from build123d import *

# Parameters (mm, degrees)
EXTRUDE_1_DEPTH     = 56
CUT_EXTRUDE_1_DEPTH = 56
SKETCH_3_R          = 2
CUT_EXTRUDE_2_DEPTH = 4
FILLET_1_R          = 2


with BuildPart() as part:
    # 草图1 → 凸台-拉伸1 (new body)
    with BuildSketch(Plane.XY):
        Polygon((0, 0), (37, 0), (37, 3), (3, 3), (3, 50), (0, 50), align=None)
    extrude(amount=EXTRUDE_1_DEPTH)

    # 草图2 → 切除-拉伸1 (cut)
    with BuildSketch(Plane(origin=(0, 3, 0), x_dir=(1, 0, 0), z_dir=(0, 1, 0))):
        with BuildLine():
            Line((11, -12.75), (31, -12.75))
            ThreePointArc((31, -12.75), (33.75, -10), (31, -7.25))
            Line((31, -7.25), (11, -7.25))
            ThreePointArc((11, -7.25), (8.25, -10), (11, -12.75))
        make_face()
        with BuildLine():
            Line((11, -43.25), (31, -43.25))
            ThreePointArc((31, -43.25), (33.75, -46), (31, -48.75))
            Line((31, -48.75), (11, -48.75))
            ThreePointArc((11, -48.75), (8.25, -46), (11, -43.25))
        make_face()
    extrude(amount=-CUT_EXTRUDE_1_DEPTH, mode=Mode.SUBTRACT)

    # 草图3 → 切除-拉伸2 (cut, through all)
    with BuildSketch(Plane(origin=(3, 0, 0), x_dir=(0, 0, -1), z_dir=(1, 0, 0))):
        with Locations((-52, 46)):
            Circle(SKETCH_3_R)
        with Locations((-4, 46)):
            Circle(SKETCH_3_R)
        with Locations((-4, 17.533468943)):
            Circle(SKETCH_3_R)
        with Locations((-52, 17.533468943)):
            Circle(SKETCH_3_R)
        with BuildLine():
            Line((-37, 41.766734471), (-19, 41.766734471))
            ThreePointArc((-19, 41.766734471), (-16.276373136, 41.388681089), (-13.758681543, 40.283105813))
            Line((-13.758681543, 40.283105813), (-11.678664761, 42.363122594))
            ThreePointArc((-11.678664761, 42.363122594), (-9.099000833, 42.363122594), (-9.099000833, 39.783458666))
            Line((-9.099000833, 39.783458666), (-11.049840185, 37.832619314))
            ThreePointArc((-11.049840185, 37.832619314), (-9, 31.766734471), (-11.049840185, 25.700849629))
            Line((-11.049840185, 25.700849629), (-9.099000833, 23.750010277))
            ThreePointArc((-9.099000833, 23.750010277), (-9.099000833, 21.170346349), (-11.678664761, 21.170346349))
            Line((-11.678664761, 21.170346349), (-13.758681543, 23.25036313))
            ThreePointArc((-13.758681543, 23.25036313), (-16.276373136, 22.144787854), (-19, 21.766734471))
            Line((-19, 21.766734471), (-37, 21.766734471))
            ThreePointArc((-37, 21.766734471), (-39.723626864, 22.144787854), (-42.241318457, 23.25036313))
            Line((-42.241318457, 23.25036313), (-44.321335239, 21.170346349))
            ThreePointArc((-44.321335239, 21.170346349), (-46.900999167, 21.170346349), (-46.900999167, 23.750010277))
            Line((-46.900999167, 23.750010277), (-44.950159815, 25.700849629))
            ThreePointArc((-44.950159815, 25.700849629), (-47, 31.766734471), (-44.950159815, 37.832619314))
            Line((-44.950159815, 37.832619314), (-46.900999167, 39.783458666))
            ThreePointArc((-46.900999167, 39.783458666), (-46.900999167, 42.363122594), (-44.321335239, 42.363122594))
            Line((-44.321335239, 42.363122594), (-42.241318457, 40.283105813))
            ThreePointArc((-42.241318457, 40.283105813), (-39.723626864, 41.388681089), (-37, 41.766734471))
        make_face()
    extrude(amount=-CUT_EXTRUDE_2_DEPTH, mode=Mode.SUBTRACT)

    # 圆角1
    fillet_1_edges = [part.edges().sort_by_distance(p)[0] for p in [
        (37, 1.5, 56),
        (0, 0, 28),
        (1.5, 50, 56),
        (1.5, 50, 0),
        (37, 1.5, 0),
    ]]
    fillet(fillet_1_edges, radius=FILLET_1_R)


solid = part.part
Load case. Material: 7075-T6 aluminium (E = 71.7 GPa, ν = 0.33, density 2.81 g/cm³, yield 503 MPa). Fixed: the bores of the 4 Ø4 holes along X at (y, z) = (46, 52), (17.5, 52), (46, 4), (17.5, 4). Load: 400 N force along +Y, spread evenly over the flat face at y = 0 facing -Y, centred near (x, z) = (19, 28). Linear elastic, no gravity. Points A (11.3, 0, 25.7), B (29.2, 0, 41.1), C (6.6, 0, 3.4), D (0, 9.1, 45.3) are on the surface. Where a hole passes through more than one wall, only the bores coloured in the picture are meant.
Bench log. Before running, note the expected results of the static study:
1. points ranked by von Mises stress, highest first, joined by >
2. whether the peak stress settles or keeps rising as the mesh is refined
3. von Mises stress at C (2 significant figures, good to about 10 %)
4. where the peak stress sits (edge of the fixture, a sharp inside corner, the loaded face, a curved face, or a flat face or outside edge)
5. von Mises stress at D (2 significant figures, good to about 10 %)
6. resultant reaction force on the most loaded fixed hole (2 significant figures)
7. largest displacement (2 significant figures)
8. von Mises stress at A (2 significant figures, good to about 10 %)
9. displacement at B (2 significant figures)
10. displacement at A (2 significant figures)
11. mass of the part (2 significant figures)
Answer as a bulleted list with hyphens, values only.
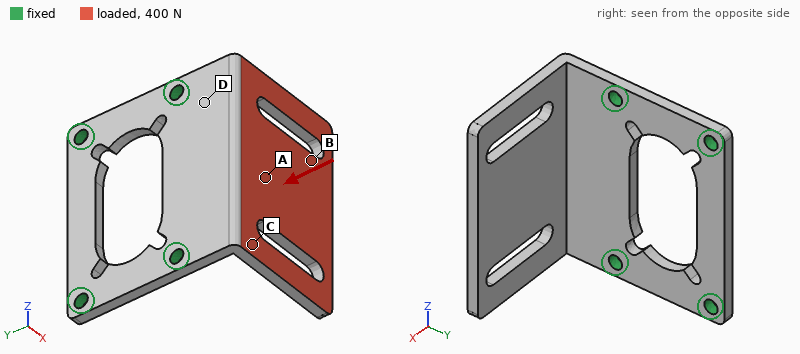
- D > C > A > B
- keeps rising
- 60 MPa
- edge of the fixture
- 81 MPa
- 210 N
- 0.82 mm
- 45 MPa
- 0.62 mm
- 0.25 mm
- 31 g
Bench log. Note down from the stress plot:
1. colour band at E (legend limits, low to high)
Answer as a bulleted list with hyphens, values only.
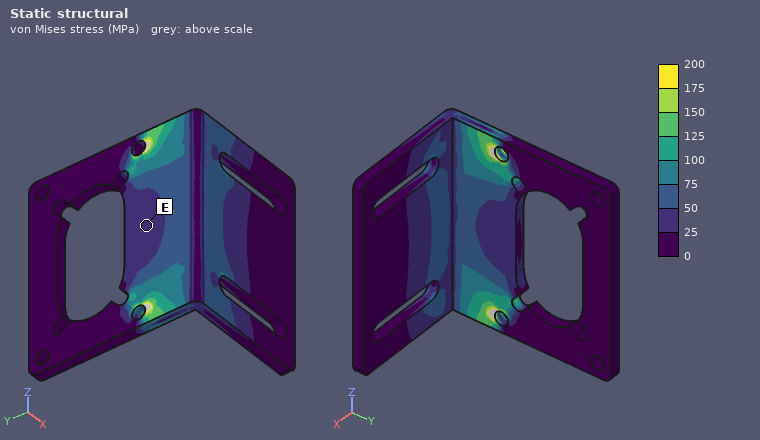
- 25 to 50 MPa
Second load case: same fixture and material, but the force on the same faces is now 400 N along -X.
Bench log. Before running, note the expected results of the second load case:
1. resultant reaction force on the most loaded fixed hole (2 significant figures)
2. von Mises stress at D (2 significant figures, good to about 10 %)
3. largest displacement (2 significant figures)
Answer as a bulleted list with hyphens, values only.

- 210 N
- 46 MPa
- 0.38 mm
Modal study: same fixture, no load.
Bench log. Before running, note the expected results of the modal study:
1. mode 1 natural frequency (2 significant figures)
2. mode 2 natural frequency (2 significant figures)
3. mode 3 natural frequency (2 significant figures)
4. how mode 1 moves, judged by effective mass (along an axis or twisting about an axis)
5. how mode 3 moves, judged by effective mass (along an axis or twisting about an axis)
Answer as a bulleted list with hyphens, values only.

- 1100 Hz
- 2500 Hz
- 3600 Hz
- along Y
- along X
